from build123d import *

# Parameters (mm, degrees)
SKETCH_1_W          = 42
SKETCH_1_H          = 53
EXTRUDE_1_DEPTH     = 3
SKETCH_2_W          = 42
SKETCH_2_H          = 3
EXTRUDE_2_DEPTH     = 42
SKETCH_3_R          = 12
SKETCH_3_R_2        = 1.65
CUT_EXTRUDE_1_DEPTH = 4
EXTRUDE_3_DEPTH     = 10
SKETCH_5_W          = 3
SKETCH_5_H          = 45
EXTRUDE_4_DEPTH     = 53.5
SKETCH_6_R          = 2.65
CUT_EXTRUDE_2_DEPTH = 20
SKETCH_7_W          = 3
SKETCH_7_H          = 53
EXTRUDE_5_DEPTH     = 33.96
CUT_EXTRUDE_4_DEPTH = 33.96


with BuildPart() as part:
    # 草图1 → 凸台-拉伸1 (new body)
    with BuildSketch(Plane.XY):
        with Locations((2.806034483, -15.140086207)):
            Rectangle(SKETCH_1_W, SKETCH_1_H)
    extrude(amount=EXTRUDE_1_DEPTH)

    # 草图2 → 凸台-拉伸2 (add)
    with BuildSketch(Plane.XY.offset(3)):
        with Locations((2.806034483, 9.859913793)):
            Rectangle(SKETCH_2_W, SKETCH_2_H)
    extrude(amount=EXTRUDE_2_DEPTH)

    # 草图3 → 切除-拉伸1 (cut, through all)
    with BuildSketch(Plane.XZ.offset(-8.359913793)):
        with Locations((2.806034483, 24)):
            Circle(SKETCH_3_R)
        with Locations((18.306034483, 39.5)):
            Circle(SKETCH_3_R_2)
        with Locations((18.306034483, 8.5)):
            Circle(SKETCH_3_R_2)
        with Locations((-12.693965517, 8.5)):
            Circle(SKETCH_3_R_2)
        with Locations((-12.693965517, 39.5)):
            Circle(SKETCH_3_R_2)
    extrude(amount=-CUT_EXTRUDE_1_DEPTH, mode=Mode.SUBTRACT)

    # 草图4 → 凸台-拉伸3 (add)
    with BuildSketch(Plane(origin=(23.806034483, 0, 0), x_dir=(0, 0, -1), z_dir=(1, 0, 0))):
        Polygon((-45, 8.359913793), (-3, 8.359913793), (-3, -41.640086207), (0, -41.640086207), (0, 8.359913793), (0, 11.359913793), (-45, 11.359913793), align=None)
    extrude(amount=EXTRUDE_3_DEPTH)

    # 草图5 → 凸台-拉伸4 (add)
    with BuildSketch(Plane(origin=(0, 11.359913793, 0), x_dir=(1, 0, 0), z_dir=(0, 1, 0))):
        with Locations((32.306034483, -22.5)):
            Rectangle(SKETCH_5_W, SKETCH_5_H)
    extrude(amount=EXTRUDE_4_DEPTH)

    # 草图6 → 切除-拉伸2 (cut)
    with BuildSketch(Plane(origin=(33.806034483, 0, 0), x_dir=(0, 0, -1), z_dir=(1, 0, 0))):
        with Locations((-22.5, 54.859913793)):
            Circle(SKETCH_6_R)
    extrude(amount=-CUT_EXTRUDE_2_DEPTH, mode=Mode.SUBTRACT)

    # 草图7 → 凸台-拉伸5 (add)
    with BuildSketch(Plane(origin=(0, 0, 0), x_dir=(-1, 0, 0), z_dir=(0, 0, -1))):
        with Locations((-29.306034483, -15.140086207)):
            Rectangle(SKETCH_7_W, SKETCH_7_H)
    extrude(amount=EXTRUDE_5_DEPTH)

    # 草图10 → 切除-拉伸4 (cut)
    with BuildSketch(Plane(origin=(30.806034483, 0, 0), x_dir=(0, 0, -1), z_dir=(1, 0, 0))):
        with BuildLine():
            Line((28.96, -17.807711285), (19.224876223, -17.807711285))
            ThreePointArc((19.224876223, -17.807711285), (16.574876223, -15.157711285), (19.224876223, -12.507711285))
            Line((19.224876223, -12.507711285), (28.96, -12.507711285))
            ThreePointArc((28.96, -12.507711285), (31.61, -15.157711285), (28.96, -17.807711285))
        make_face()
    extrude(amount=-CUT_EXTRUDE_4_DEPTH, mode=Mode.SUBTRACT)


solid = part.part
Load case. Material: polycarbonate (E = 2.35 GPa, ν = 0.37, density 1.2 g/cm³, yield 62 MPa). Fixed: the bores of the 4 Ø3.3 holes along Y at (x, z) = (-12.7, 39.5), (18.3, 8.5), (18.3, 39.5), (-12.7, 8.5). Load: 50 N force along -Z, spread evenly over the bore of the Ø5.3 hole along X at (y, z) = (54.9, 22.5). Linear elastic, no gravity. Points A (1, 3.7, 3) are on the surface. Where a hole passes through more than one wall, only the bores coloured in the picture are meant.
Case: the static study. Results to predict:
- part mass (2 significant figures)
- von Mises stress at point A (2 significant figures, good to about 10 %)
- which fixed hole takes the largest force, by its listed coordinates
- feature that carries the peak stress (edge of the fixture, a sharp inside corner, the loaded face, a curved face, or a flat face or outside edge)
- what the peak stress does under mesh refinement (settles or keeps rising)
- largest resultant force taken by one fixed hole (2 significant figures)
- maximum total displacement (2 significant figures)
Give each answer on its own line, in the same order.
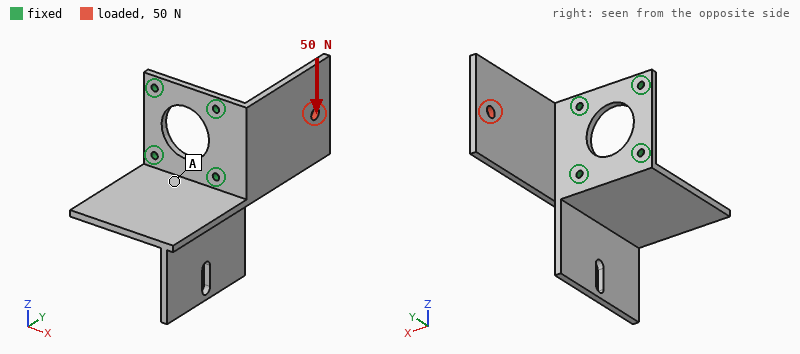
31 g
1.7 MPa
(18.3, 8.5)
edge of the fixture
keeps rising
87 N
1.5 mm
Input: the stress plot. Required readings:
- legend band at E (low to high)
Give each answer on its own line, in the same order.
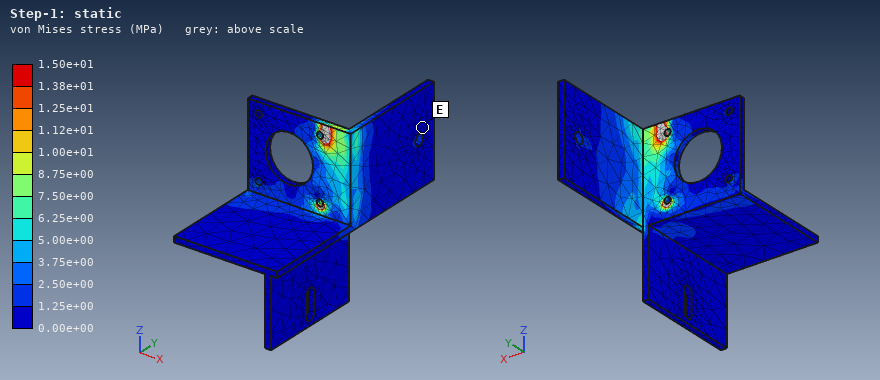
0.00e+00 to 1.25e+00 MPa
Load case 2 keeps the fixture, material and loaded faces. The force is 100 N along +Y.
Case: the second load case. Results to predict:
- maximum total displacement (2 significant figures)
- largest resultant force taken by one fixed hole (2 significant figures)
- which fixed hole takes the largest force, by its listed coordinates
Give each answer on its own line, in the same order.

1.5 mm
73 N
(18.3, 8.5)
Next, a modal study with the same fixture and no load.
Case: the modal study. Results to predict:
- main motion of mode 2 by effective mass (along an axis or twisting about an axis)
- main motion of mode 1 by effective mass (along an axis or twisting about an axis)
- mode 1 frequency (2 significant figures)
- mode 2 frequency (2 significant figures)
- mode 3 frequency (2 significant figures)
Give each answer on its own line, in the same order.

along Z
along X
190 Hz
210 Hz
350 Hz
